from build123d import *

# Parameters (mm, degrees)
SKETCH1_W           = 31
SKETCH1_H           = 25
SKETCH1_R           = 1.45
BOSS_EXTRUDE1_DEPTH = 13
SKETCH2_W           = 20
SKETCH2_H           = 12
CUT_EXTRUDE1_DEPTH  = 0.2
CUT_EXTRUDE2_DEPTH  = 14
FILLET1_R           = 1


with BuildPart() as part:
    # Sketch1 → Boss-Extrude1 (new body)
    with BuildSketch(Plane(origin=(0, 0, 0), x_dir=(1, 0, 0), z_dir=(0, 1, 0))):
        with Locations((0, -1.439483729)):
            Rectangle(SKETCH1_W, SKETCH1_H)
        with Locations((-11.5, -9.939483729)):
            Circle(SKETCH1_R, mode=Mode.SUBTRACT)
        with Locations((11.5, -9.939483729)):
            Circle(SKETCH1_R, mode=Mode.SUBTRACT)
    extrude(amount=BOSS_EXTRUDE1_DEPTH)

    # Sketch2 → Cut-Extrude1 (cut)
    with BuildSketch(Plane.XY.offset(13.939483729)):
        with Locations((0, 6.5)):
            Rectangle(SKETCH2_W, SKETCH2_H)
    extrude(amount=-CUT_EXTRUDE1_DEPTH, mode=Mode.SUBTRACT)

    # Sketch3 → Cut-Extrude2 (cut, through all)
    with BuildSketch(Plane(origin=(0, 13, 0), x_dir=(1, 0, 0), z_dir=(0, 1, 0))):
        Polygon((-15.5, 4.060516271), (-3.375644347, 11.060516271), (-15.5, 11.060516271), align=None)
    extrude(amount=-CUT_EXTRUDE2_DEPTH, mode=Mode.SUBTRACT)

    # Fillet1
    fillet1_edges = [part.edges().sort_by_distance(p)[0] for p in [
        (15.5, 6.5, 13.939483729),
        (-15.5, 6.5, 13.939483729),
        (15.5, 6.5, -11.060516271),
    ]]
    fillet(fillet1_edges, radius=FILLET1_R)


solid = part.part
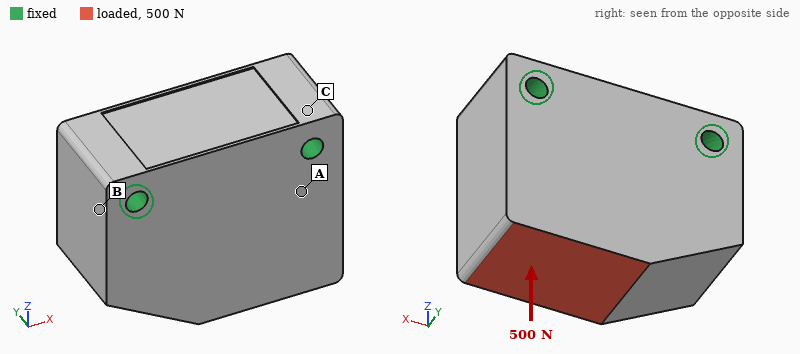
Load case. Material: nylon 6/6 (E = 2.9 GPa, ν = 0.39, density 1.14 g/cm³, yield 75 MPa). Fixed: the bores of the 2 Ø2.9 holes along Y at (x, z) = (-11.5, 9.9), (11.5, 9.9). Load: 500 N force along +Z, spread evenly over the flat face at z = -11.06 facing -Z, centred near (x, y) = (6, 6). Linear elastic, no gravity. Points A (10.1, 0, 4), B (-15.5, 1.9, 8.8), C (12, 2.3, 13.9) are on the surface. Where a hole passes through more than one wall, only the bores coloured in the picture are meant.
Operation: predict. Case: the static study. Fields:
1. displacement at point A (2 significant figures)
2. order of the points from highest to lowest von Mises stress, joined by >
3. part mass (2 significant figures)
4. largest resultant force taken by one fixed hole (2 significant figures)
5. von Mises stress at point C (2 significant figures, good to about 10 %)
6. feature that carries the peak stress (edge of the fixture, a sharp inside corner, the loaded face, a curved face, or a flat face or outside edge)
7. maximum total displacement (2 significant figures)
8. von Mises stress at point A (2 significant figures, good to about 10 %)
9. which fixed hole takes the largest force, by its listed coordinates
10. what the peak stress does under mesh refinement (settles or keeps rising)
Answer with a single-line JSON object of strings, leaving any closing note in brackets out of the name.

{"displacement at point A": "6.5 µm", "order of the points from highest to lowest von Mises stress, joined by >": "A > C > B", "part mass": "11 g", "largest resultant force taken by one fixed hole": "370 N", "von Mises stress at point C": "1.7 MPa", "feature that carries the peak stress": "edge of the fixture", "maximum total displacement": "19 µm", "von Mises stress at point A": "2.9 MPa", "which fixed hole takes the largest force, by its listed coordinates": "(11.5, 9.9)", "what the peak stress does under mesh refinement": "keeps rising"}
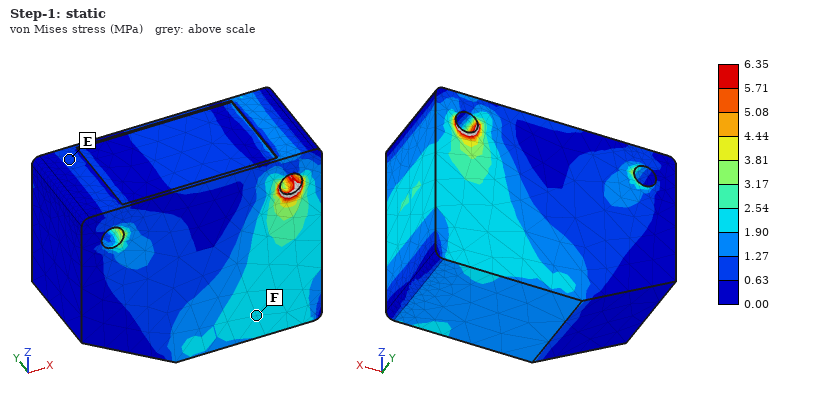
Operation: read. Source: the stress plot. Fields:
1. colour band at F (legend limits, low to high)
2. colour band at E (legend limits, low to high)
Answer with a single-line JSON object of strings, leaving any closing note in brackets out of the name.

{"colour band at F": "1.90 to 2.54 MPa", "colour band at E": "0.63 to 1.27 MPa"}
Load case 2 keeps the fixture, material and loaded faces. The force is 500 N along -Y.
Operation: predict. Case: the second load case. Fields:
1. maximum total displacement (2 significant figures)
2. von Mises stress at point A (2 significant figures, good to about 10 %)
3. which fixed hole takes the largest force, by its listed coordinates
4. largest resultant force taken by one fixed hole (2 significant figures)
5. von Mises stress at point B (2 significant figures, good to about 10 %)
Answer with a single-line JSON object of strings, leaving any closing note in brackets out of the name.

{"maximum total displacement": "0.23 mm", "von Mises stress at point A": "14 MPa", "which fixed hole takes the largest force, by its listed coordinates": "(11.5, 9.9)", "largest resultant force taken by one fixed hole": "350 N", "von Mises stress at point B": "6.1 MPa"}
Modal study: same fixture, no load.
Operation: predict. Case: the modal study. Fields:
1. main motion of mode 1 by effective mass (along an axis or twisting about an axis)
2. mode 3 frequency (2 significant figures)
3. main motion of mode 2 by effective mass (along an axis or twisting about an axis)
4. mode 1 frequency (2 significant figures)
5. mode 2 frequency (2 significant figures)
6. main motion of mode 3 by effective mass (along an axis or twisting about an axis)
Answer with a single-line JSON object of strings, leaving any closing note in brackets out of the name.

{"main motion of mode 1 by effective mass": "along Y", "mode 3 frequency": "10 kHz", "main motion of mode 2 by effective mass": "along X", "mode 1 frequency": "5200 Hz", "mode 2 frequency": "9300 Hz", "main motion of mode 3 by effective mass": "twisting about Z"}
